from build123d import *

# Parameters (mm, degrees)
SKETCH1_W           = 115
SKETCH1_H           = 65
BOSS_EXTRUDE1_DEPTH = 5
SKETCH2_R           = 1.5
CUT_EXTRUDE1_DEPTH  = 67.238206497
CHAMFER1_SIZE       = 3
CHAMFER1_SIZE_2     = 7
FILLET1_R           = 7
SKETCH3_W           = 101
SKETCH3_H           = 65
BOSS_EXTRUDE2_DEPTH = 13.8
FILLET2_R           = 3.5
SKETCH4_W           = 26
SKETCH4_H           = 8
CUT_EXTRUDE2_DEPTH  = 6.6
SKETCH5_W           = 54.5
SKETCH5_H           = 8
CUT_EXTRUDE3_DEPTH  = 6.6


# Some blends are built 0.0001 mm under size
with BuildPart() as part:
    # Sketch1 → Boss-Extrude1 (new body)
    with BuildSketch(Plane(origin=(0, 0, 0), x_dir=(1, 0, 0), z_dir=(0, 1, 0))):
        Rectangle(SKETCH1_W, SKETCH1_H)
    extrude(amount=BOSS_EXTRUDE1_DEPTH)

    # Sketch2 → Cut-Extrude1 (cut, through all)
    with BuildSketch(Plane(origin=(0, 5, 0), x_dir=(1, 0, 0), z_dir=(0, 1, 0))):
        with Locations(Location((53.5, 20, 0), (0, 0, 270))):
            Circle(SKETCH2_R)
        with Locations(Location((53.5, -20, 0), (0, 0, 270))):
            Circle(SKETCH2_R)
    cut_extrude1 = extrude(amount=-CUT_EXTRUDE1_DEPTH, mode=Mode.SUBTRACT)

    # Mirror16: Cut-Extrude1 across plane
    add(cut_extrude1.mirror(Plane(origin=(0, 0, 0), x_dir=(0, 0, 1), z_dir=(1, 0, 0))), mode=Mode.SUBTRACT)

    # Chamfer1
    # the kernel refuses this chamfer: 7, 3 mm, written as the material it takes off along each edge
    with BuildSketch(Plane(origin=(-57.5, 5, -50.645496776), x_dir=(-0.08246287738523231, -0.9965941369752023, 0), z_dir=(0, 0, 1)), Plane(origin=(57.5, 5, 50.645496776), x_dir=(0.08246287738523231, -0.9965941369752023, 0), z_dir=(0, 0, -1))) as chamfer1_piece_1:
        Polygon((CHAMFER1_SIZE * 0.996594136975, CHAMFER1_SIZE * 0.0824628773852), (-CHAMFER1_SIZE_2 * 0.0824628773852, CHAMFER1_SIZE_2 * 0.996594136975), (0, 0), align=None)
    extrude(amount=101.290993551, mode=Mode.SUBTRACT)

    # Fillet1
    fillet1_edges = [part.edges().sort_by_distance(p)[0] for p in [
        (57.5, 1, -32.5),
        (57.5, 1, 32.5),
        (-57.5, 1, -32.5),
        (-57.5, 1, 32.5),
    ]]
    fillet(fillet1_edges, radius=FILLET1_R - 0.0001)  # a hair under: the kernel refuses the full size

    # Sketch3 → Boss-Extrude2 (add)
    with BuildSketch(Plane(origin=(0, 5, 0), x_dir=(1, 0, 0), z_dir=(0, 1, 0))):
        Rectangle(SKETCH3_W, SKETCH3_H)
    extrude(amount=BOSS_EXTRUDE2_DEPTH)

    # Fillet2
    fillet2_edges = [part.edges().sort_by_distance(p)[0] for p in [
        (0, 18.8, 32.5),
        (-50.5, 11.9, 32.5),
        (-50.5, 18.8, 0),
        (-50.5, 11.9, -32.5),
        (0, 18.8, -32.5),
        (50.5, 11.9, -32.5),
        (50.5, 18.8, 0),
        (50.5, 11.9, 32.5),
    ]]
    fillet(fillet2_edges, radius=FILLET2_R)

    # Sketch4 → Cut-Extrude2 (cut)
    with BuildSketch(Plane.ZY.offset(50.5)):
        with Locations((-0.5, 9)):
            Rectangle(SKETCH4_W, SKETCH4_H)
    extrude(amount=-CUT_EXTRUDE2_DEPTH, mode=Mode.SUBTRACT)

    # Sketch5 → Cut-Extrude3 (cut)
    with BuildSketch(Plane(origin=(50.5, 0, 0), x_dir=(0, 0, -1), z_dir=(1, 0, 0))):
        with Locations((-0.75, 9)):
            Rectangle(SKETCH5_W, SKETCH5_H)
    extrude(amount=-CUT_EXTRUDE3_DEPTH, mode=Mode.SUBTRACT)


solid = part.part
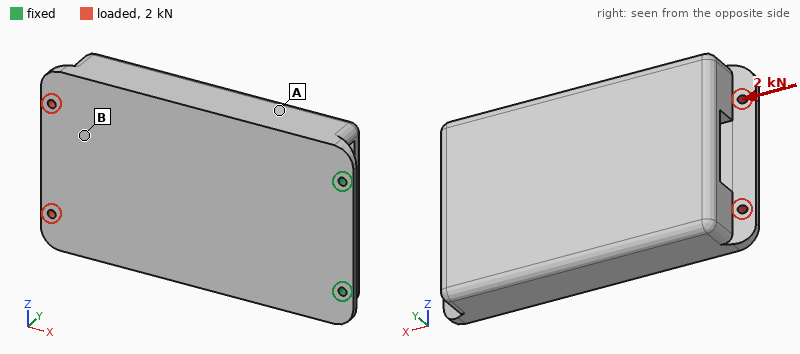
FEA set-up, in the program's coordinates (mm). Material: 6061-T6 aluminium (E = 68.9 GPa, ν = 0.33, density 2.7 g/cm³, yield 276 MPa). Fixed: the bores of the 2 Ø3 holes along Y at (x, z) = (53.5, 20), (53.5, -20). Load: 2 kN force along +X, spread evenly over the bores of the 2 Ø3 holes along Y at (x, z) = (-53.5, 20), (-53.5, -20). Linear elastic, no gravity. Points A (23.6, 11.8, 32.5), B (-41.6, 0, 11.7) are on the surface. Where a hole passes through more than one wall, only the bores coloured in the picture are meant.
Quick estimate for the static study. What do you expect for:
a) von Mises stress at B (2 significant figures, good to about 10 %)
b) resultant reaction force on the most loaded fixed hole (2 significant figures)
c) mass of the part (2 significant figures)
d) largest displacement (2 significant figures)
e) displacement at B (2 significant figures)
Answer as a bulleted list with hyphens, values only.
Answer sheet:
- 8.2 MPa
- 1.0 kN
- 330 g
- 83 µm
- 63 µm
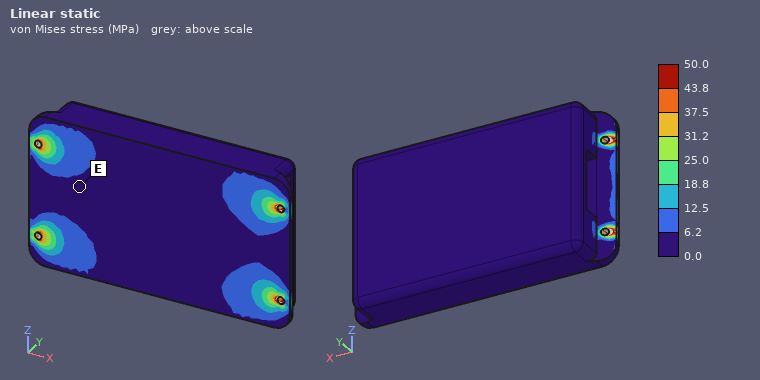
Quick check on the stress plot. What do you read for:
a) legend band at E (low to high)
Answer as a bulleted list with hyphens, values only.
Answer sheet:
- 0.0 to 6.2 MPa
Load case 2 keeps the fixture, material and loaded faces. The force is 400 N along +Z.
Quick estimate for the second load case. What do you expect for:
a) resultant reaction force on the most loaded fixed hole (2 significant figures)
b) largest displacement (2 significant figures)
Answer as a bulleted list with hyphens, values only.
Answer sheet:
- 1.1 kN
- 35 µm
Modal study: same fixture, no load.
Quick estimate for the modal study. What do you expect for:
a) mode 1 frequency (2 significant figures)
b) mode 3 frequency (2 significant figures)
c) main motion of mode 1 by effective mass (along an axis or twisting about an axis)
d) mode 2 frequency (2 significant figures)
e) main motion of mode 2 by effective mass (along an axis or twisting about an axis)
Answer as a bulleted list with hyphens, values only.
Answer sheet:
- 210 Hz
- 2400 Hz
- along Y
- 1800 Hz
- along Z
